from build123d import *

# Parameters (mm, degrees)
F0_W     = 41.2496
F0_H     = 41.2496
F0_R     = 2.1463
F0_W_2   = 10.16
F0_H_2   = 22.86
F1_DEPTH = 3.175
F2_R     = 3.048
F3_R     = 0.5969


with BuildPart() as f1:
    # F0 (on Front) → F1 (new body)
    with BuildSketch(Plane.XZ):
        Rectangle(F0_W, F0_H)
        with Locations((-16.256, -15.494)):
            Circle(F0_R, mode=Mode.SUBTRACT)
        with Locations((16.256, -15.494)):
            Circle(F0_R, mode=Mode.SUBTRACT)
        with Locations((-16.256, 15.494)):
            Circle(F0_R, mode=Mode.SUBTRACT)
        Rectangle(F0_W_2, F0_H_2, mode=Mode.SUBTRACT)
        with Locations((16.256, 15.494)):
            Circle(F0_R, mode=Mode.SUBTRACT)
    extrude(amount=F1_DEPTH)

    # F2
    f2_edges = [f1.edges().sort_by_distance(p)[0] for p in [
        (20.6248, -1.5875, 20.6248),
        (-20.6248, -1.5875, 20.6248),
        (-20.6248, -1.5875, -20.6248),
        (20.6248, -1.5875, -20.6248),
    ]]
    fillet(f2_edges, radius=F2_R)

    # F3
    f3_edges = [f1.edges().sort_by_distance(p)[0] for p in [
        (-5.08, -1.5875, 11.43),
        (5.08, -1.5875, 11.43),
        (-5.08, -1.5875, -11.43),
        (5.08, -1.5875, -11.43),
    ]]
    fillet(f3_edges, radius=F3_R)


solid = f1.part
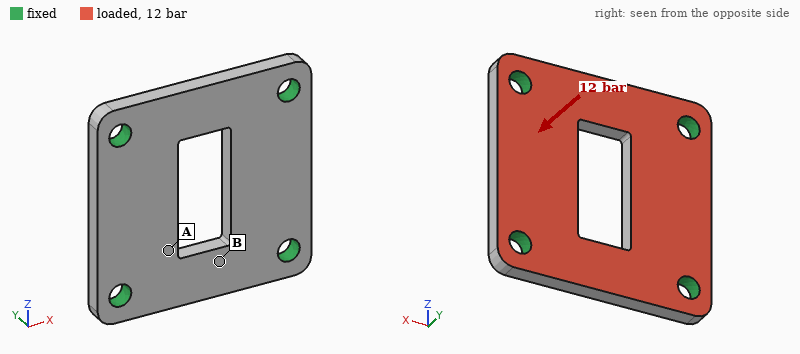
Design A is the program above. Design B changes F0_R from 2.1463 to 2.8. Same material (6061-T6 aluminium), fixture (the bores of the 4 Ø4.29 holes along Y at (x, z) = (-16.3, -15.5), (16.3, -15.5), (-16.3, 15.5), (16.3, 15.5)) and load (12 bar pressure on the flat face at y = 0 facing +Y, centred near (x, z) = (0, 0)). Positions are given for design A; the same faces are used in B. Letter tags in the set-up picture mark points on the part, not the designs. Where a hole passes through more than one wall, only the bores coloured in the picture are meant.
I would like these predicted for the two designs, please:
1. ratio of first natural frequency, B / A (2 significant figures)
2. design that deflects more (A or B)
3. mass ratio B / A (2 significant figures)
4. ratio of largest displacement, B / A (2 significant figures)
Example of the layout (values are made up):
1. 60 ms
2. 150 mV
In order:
1. 1.1
2. A
3. 0.97
4. 0.80
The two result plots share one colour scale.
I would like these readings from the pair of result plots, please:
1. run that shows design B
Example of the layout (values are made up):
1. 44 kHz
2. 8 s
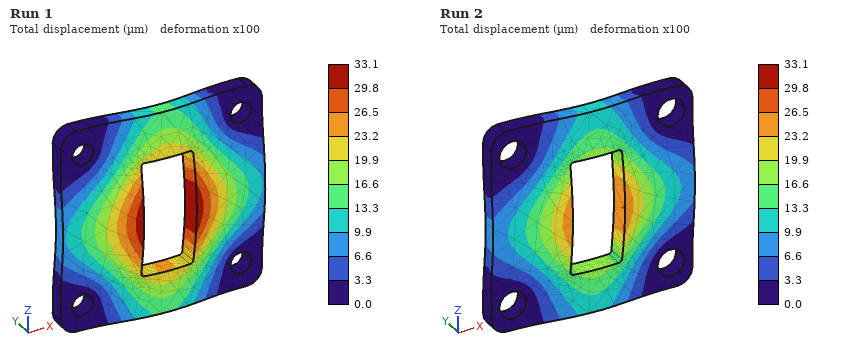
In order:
1. Run 2
